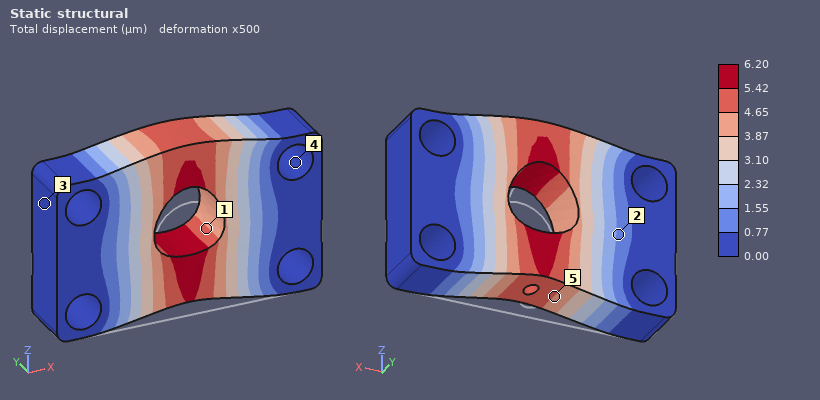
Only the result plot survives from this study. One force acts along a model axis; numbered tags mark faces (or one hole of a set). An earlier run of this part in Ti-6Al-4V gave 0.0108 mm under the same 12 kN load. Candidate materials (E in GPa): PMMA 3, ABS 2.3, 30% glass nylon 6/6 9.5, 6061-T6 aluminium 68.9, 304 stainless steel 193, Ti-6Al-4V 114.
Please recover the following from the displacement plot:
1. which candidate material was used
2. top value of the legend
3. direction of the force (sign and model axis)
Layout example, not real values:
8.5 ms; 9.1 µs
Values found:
304 stainless steel; 6.20 µm; +Z
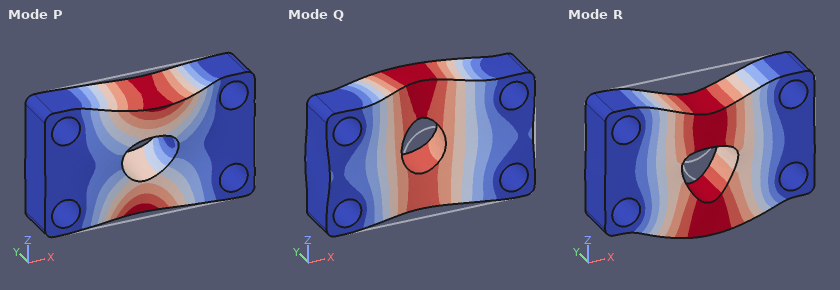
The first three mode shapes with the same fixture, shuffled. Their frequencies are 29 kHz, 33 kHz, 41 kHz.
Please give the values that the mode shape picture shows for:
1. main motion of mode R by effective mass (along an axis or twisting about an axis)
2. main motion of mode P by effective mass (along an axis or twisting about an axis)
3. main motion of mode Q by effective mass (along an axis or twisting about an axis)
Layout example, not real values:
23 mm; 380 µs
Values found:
along Z; twisting about X; along Y
